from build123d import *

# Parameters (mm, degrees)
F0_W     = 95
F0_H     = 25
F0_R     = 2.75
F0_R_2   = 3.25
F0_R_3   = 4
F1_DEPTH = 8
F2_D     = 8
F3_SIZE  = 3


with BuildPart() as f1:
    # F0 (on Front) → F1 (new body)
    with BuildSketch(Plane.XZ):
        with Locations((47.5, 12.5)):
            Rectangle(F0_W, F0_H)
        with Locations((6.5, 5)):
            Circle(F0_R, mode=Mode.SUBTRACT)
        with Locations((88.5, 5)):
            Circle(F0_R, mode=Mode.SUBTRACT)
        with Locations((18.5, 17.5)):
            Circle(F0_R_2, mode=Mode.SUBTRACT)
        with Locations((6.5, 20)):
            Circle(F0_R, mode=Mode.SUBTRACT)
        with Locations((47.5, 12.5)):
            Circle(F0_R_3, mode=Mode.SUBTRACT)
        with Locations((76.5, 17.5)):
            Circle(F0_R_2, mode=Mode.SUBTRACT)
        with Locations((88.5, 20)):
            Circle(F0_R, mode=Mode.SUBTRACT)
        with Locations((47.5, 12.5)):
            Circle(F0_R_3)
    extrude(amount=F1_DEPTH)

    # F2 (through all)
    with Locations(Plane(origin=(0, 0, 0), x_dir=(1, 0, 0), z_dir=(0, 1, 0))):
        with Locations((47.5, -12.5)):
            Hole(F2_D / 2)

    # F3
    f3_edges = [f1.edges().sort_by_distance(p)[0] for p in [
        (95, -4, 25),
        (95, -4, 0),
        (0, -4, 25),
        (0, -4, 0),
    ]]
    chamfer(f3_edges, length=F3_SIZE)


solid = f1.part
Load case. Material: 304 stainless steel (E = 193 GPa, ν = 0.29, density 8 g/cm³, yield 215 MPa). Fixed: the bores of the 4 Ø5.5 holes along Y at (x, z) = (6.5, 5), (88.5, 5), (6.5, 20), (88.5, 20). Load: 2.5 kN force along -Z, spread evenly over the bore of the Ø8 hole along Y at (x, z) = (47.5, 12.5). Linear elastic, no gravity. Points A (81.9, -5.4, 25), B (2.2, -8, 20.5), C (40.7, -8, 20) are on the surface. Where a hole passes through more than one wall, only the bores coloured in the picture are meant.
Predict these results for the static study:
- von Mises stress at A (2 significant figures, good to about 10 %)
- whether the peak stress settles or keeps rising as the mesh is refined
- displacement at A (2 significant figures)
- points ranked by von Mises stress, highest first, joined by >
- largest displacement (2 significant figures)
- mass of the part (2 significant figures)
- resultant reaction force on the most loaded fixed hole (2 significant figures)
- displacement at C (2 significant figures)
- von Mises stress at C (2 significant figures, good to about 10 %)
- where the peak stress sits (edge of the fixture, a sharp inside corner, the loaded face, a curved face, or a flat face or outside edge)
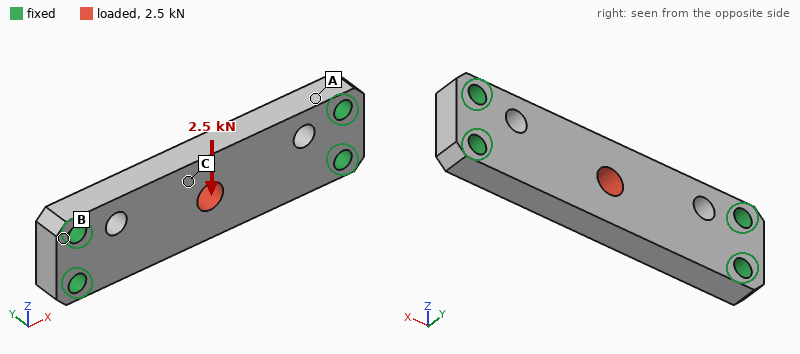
27 MPa
keeps rising
1.2 µm
A > C > B
7.9 µm
140 g
1.5 kN
7.0 µm
17 MPa
edge of the fixture
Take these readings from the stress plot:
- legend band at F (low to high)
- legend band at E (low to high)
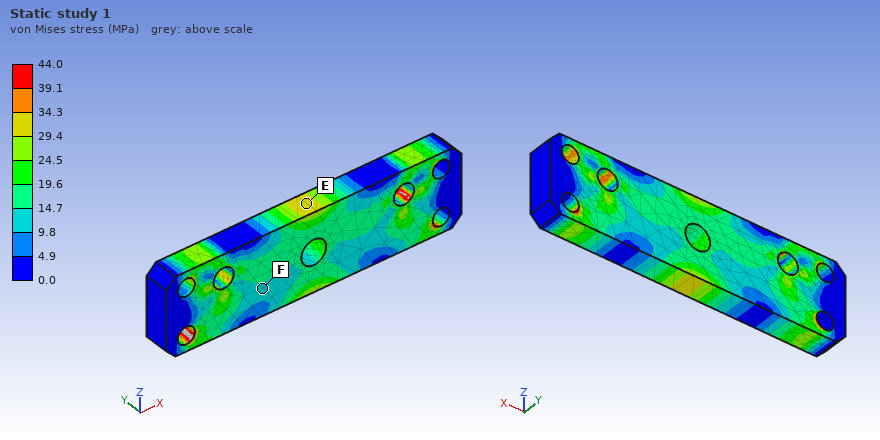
9.8 to 14.7 MPa
29.4 to 34.3 MPa
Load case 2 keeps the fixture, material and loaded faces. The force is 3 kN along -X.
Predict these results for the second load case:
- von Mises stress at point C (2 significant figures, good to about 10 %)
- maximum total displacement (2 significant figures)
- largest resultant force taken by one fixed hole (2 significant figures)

7.0 MPa
2.0 µm
850 N
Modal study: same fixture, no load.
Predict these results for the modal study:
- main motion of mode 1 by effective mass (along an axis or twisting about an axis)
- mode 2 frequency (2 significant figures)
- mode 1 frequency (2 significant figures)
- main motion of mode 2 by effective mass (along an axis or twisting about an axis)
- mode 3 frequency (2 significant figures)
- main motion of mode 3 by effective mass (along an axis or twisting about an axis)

along Y
11 kHz
5900 Hz
twisting about X
13 kHz
along Z
